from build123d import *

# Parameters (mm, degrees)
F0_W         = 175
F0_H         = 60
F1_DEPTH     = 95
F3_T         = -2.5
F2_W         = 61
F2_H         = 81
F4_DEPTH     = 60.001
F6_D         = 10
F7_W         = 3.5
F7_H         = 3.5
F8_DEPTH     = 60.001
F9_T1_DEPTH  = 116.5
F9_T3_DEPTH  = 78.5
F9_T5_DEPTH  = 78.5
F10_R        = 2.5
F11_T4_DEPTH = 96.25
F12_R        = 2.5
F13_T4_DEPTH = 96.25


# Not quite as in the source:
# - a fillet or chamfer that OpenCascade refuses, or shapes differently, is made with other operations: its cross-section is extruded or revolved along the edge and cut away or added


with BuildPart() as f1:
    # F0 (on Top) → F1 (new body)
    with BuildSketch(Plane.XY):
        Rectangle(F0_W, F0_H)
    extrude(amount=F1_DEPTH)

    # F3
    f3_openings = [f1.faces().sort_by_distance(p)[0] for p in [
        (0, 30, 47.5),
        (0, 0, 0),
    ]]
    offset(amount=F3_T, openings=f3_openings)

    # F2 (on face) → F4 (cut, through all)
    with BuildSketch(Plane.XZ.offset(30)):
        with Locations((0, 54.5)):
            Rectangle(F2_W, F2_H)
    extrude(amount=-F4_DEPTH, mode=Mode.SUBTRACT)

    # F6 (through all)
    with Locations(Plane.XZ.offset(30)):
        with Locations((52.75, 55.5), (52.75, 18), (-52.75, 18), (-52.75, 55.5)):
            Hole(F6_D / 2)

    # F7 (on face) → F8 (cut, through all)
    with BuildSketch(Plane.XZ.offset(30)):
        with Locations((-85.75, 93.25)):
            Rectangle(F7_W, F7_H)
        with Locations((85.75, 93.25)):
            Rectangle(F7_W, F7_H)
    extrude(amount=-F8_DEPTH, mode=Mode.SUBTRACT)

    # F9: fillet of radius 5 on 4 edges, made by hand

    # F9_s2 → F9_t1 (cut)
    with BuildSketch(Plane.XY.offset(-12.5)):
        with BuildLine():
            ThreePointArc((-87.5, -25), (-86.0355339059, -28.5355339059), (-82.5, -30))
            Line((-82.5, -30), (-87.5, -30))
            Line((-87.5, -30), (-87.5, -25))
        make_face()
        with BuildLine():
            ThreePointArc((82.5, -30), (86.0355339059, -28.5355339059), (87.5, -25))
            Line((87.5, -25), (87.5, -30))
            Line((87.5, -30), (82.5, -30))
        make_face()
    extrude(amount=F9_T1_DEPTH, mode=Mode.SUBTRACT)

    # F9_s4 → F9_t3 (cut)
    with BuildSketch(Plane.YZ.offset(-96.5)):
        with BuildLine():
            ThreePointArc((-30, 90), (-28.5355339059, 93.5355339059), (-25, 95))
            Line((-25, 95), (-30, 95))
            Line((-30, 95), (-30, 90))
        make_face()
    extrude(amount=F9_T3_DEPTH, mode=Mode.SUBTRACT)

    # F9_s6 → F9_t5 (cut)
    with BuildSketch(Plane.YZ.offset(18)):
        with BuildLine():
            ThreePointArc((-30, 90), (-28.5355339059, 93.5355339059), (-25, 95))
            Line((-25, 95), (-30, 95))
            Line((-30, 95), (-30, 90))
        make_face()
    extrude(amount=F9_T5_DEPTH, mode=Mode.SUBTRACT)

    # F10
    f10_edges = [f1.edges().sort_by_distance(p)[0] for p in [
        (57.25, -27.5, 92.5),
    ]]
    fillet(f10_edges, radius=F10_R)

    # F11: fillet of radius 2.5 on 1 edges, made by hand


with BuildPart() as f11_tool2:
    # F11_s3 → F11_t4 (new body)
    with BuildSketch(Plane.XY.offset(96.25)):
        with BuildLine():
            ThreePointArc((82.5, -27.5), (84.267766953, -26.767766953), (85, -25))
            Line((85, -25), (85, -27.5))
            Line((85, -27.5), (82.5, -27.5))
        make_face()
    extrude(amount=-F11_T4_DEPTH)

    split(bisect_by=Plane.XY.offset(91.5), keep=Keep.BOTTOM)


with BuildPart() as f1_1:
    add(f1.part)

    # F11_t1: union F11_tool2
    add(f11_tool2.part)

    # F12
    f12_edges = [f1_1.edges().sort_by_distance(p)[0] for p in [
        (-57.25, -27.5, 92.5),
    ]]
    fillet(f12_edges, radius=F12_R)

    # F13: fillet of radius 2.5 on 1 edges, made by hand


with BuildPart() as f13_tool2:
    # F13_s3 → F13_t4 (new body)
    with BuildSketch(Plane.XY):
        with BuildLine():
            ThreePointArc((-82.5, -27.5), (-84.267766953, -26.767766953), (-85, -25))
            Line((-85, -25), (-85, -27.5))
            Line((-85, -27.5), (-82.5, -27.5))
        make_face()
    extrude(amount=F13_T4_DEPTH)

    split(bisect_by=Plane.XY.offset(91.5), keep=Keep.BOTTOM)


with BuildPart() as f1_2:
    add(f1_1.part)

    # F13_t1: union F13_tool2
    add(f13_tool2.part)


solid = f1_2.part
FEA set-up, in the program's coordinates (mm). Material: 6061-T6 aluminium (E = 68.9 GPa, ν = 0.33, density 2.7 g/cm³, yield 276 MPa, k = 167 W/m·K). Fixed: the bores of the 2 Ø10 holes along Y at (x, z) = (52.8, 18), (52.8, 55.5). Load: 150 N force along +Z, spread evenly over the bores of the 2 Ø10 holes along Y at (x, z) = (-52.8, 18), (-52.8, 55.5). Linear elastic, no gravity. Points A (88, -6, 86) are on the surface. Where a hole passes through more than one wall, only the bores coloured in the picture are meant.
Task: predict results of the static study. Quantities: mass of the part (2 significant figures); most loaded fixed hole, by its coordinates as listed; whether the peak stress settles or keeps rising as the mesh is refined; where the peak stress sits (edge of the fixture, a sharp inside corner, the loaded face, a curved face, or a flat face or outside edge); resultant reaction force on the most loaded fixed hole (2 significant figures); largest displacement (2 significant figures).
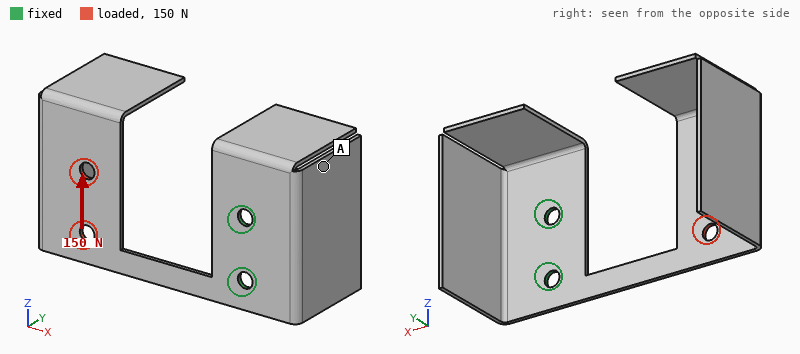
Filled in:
190 g
(52.8, 55.5)
keeps rising
a sharp inside corner
350 N
2.0 mm
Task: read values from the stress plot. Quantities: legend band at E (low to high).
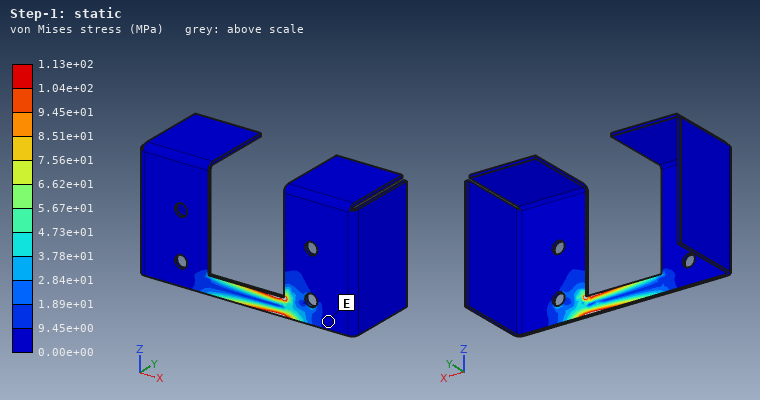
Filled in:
0.00e+00 to 9.45e+00 MPa
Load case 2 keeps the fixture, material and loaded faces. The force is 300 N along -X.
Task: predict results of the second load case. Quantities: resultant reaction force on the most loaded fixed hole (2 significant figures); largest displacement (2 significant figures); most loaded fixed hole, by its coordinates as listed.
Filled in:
210 N
2.1 mm
(52.8, 18)
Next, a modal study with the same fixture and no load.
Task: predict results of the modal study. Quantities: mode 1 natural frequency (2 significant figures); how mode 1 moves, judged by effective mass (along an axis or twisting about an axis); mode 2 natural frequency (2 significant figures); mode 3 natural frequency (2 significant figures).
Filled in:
23 Hz
along Y
53 Hz
140 Hz
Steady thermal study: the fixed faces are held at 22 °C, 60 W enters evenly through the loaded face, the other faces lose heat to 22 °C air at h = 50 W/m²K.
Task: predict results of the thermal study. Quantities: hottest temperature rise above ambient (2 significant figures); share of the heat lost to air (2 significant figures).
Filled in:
76 K
95 %
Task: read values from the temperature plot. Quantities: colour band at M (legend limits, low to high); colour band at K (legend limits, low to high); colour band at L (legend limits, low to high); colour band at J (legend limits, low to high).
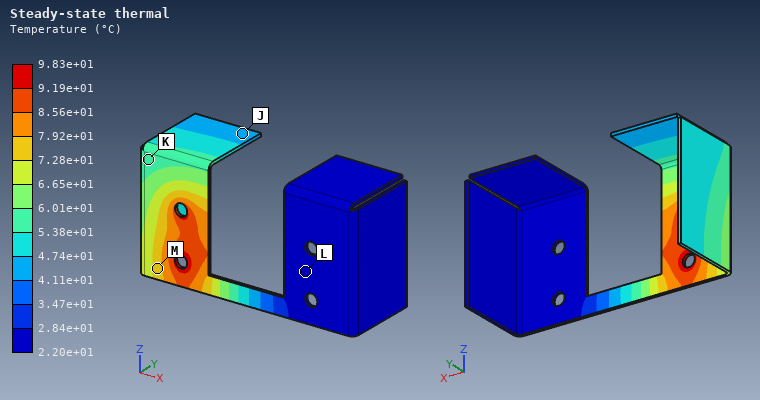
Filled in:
7.28e+01 to 7.92e+01 °C
5.38e+01 to 6.01e+01 °C
2.20e+01 to 2.84e+01 °C
4.11e+01 to 4.74e+01 °C
